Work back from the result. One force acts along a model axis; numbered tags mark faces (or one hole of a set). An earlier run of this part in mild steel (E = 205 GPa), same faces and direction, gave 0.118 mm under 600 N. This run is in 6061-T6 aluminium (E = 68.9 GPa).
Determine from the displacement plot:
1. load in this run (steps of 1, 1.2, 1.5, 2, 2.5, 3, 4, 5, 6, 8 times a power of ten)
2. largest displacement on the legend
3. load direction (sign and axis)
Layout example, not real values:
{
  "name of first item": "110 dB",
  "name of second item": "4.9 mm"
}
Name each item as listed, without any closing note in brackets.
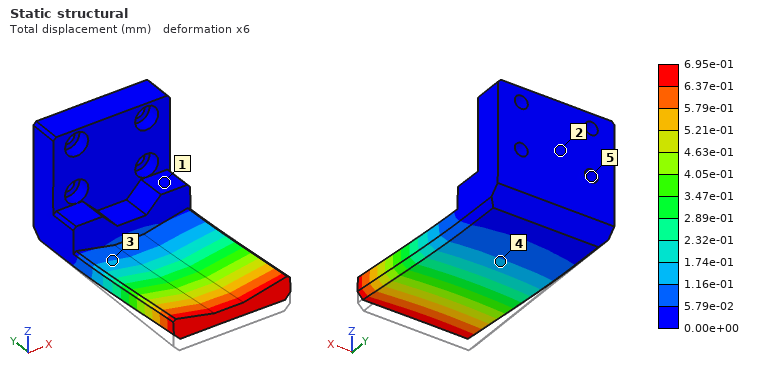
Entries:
{
  "load in this run": "1.2 kN",
  "largest displacement on the legend": "6.95e-01 mm",
  "load direction": "+Z"
}
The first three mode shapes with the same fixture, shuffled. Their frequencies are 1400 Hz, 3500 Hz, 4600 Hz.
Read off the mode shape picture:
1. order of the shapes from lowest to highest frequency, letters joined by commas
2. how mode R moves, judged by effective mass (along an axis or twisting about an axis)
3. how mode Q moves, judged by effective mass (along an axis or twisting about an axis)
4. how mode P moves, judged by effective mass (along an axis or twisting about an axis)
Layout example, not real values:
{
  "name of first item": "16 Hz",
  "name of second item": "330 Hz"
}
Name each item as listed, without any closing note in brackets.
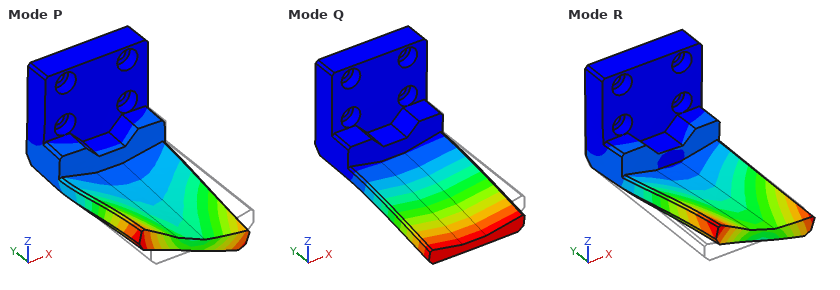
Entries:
{
  "order of the shapes from lowest to highest frequency, letters joined by commas": "Q, R, P",
  "how mode R moves, judged by effective mass": "along X",
  "how mode Q moves, judged by effective mass": "along Z",
  "how mode P moves, judged by effective mass": "along X"
}
